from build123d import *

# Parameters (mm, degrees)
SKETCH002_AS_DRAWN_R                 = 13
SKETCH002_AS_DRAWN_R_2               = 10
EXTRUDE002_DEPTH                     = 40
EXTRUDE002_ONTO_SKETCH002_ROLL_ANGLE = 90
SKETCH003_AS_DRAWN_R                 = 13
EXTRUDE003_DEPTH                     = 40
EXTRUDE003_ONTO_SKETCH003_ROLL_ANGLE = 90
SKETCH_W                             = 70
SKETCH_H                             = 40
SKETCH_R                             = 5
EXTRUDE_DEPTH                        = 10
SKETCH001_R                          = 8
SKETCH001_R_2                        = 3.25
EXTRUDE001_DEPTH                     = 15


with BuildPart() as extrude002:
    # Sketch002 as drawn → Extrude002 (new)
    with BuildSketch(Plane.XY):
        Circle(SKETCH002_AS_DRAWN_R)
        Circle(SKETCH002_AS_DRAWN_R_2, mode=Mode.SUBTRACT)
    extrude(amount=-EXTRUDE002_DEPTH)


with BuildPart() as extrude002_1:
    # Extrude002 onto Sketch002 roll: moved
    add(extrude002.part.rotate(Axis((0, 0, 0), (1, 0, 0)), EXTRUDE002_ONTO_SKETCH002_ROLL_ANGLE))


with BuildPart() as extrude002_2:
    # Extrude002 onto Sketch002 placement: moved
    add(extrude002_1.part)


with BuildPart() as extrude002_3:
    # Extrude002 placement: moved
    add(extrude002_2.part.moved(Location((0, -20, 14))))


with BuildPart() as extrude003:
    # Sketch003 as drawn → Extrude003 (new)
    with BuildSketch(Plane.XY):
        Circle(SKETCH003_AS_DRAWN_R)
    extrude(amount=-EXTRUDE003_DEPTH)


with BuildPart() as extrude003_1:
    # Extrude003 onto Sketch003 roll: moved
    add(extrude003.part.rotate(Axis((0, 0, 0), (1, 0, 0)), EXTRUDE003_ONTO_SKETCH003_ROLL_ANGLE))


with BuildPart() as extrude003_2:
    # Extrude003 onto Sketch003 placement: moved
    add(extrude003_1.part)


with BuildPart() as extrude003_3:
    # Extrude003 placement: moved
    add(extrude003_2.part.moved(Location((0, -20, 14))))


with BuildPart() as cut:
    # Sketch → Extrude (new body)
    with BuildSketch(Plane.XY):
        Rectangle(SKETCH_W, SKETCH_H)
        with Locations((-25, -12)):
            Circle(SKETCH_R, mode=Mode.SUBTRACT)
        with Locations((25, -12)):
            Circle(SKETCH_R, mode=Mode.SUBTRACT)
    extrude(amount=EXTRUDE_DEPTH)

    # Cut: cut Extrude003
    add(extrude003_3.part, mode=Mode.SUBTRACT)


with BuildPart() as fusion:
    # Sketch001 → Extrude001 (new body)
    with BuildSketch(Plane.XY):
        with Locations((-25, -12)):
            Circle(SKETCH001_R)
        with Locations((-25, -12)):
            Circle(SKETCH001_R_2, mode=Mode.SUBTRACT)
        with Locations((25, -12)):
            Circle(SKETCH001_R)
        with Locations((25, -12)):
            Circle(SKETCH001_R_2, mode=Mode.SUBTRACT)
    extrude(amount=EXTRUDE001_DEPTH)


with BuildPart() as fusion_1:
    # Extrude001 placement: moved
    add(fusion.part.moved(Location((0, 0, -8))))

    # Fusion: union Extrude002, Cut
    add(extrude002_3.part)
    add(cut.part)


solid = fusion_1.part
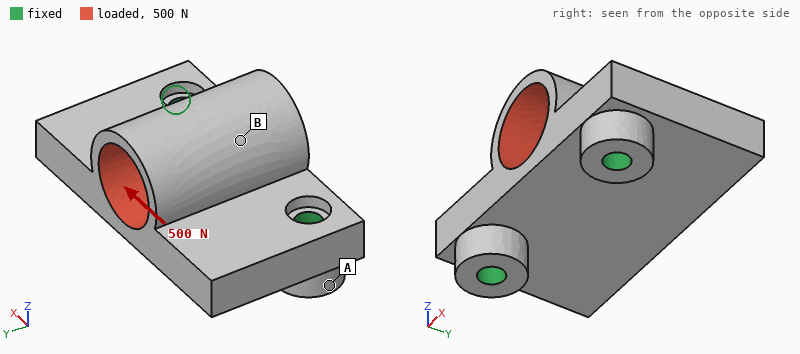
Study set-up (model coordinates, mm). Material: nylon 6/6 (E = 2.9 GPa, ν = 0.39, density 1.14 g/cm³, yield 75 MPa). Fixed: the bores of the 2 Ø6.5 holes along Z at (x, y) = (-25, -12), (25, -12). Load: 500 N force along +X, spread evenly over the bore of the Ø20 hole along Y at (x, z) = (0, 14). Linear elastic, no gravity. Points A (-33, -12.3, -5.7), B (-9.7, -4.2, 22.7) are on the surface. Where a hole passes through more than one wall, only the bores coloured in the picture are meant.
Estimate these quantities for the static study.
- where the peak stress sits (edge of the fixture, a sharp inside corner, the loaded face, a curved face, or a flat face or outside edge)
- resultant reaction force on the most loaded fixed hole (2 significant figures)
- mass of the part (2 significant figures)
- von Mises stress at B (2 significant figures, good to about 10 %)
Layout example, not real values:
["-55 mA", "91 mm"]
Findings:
["the loaded face", "290 N", "36 g", "5.1 MPa"]
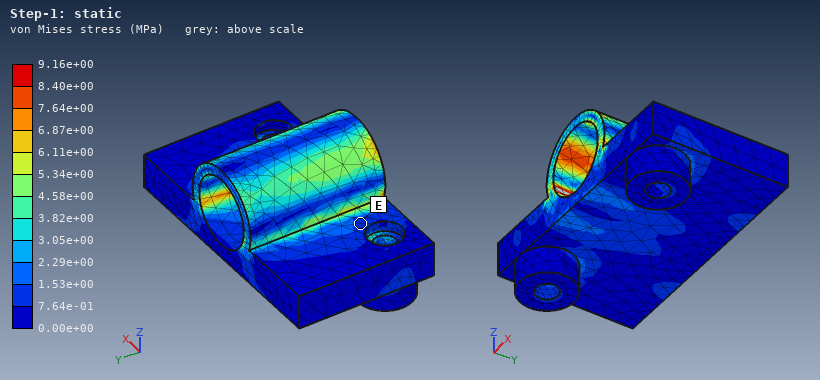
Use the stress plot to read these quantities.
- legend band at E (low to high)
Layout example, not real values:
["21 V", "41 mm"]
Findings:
["7.64e-01 to 1.53e+00 MPa"]
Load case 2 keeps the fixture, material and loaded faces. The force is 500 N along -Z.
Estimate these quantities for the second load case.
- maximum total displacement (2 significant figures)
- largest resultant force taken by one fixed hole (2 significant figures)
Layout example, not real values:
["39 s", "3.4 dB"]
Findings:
["0.21 mm", "250 N"]
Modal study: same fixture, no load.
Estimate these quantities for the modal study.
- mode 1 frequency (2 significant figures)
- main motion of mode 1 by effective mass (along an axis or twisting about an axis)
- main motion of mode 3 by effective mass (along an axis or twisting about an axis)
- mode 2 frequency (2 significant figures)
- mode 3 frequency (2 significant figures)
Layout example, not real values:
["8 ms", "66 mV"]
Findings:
["1800 Hz", "along Z", "along X", "3100 Hz", "3800 Hz"]
